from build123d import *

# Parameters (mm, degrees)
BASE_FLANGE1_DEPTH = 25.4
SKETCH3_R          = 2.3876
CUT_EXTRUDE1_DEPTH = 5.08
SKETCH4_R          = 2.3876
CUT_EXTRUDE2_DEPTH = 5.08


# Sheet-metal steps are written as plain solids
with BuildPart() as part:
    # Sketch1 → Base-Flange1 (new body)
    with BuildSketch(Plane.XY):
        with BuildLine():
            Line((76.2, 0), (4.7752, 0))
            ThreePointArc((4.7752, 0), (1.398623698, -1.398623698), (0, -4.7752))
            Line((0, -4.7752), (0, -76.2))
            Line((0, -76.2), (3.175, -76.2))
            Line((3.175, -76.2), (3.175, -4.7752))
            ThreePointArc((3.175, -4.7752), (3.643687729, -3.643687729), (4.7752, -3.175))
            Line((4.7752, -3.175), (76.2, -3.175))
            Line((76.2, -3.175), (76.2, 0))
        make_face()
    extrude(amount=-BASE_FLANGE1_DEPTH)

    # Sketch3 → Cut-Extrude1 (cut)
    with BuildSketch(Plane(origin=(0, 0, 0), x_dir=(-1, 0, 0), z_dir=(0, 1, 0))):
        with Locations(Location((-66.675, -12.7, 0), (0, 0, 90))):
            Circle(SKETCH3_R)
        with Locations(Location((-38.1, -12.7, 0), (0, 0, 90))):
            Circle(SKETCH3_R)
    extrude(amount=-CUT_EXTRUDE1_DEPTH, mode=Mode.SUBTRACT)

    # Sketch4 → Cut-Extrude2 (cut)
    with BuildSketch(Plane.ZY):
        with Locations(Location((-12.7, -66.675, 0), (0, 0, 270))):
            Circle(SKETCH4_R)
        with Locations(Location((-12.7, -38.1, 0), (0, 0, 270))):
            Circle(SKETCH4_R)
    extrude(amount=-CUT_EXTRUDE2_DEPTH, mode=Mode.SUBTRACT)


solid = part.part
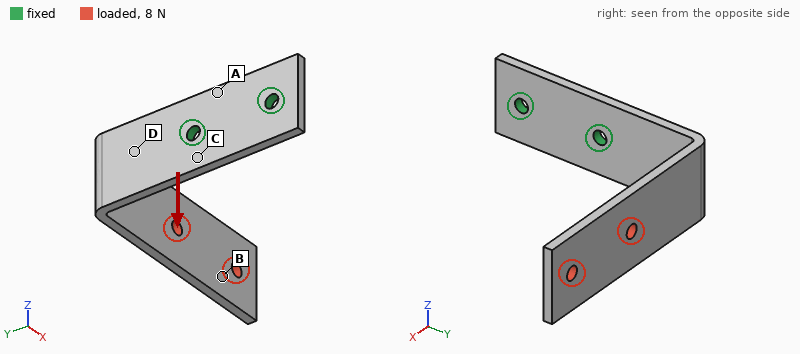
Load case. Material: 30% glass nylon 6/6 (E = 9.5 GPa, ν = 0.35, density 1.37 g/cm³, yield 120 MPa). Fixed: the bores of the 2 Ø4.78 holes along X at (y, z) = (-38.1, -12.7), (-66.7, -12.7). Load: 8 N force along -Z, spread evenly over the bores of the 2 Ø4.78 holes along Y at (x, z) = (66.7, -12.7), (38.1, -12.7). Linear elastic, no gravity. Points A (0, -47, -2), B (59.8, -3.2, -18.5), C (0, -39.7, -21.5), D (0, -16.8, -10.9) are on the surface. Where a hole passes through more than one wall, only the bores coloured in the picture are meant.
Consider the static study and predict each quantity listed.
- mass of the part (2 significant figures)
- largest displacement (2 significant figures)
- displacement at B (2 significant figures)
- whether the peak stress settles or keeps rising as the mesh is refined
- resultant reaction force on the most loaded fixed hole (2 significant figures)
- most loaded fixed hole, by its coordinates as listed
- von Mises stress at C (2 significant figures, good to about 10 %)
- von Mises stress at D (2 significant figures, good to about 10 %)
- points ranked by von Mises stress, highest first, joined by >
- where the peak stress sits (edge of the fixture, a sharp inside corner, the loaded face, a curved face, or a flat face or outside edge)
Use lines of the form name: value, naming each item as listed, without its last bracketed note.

mass of the part: 16 g
largest displacement: 1.1 mm
displacement at B: 0.88 mm
whether the peak stress settles or keeps rising as the mesh is refined: keeps rising
resultant reaction force on the most loaded fixed hole: 16 N
most loaded fixed hole, by its coordinates as listed: (-38.1, -12.7)
von Mises stress at C: 5.3 MPa
von Mises stress at D: 8.1 MPa
points ranked by von Mises stress, highest first, joined by >: D > C > A > B
where the peak stress sits: edge of the fixture
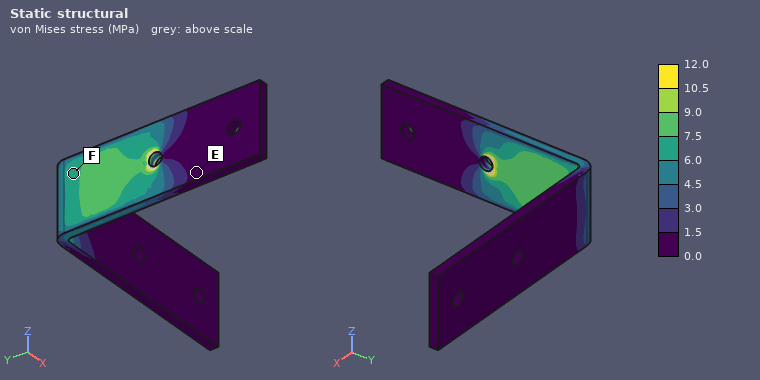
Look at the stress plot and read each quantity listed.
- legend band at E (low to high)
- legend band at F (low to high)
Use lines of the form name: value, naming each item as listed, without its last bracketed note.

legend band at E: 0.0 to 1.5 MPa
legend band at F: 6.0 to 7.5 MPa
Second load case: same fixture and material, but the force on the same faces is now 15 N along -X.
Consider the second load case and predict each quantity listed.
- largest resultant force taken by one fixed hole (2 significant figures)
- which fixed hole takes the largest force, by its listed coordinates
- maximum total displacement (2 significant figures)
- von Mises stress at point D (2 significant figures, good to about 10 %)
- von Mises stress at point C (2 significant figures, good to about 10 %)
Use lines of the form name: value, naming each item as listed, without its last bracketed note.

largest resultant force taken by one fixed hole: 18 N
which fixed hole takes the largest force, by its listed coordinates: (-38.1, -12.7)
maximum total displacement: 1.2 mm
von Mises stress at point D: 4.9 MPa
von Mises stress at point C: 3.8 MPa
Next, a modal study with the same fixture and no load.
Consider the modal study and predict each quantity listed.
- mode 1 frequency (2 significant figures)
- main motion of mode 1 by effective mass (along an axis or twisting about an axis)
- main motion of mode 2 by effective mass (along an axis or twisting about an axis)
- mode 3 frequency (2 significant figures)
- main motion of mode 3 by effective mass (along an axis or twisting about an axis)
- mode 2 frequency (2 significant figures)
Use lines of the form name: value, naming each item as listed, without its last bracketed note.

mode 1 frequency: 140 Hz
main motion of mode 1 by effective mass: along Y
main motion of mode 2 by effective mass: along Z
mode 3 frequency: 500 Hz
main motion of mode 3 by effective mass: along X
mode 2 frequency: 210 Hz
